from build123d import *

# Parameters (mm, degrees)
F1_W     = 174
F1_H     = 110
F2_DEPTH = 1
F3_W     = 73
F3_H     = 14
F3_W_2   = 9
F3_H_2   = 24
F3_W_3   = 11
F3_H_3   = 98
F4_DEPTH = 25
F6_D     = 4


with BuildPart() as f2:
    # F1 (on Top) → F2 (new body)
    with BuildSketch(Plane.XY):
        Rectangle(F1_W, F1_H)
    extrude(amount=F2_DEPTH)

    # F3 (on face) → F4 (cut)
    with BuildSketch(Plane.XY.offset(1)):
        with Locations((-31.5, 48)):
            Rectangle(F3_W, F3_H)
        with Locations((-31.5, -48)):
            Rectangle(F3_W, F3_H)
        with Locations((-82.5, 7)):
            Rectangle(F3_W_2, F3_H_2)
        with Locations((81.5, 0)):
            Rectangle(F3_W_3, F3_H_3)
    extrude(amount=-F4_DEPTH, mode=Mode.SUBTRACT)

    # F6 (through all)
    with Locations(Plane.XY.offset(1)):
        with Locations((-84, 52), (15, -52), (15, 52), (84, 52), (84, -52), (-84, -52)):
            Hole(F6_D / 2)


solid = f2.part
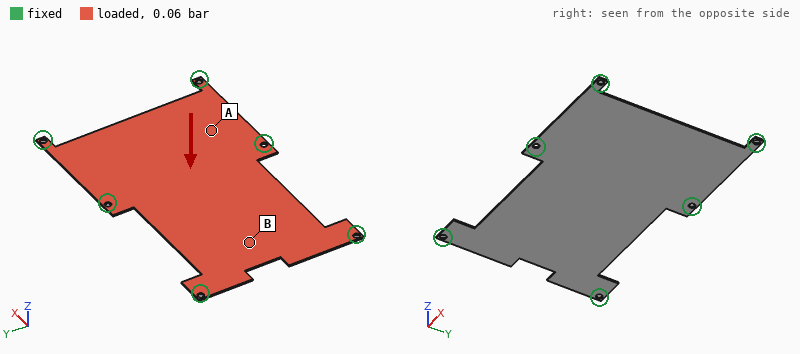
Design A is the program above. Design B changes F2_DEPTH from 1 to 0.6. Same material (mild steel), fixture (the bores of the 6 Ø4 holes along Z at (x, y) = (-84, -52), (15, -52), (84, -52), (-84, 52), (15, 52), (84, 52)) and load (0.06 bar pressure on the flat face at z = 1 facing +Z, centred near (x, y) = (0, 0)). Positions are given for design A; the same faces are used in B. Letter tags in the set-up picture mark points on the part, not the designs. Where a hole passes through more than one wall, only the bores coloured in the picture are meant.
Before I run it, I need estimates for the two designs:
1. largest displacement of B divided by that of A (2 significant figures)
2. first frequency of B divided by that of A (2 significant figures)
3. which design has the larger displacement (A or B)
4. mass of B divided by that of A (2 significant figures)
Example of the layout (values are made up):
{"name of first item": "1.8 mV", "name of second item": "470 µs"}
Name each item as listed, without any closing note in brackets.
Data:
{"largest displacement of B divided by that of A": "4.6", "first frequency of B divided by that of A": "0.60", "which design has the larger displacement": "B", "mass of B divided by that of A": "0.60"}
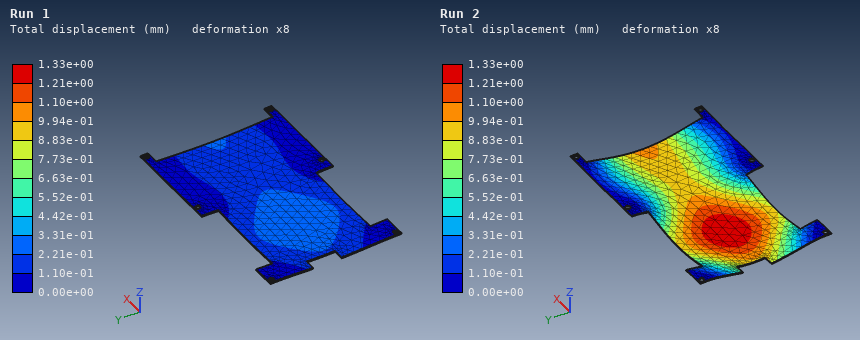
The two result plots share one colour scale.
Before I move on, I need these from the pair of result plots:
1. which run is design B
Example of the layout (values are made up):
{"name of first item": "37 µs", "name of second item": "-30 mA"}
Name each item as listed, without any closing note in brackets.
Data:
{"which run is design B": "Run 2"}
